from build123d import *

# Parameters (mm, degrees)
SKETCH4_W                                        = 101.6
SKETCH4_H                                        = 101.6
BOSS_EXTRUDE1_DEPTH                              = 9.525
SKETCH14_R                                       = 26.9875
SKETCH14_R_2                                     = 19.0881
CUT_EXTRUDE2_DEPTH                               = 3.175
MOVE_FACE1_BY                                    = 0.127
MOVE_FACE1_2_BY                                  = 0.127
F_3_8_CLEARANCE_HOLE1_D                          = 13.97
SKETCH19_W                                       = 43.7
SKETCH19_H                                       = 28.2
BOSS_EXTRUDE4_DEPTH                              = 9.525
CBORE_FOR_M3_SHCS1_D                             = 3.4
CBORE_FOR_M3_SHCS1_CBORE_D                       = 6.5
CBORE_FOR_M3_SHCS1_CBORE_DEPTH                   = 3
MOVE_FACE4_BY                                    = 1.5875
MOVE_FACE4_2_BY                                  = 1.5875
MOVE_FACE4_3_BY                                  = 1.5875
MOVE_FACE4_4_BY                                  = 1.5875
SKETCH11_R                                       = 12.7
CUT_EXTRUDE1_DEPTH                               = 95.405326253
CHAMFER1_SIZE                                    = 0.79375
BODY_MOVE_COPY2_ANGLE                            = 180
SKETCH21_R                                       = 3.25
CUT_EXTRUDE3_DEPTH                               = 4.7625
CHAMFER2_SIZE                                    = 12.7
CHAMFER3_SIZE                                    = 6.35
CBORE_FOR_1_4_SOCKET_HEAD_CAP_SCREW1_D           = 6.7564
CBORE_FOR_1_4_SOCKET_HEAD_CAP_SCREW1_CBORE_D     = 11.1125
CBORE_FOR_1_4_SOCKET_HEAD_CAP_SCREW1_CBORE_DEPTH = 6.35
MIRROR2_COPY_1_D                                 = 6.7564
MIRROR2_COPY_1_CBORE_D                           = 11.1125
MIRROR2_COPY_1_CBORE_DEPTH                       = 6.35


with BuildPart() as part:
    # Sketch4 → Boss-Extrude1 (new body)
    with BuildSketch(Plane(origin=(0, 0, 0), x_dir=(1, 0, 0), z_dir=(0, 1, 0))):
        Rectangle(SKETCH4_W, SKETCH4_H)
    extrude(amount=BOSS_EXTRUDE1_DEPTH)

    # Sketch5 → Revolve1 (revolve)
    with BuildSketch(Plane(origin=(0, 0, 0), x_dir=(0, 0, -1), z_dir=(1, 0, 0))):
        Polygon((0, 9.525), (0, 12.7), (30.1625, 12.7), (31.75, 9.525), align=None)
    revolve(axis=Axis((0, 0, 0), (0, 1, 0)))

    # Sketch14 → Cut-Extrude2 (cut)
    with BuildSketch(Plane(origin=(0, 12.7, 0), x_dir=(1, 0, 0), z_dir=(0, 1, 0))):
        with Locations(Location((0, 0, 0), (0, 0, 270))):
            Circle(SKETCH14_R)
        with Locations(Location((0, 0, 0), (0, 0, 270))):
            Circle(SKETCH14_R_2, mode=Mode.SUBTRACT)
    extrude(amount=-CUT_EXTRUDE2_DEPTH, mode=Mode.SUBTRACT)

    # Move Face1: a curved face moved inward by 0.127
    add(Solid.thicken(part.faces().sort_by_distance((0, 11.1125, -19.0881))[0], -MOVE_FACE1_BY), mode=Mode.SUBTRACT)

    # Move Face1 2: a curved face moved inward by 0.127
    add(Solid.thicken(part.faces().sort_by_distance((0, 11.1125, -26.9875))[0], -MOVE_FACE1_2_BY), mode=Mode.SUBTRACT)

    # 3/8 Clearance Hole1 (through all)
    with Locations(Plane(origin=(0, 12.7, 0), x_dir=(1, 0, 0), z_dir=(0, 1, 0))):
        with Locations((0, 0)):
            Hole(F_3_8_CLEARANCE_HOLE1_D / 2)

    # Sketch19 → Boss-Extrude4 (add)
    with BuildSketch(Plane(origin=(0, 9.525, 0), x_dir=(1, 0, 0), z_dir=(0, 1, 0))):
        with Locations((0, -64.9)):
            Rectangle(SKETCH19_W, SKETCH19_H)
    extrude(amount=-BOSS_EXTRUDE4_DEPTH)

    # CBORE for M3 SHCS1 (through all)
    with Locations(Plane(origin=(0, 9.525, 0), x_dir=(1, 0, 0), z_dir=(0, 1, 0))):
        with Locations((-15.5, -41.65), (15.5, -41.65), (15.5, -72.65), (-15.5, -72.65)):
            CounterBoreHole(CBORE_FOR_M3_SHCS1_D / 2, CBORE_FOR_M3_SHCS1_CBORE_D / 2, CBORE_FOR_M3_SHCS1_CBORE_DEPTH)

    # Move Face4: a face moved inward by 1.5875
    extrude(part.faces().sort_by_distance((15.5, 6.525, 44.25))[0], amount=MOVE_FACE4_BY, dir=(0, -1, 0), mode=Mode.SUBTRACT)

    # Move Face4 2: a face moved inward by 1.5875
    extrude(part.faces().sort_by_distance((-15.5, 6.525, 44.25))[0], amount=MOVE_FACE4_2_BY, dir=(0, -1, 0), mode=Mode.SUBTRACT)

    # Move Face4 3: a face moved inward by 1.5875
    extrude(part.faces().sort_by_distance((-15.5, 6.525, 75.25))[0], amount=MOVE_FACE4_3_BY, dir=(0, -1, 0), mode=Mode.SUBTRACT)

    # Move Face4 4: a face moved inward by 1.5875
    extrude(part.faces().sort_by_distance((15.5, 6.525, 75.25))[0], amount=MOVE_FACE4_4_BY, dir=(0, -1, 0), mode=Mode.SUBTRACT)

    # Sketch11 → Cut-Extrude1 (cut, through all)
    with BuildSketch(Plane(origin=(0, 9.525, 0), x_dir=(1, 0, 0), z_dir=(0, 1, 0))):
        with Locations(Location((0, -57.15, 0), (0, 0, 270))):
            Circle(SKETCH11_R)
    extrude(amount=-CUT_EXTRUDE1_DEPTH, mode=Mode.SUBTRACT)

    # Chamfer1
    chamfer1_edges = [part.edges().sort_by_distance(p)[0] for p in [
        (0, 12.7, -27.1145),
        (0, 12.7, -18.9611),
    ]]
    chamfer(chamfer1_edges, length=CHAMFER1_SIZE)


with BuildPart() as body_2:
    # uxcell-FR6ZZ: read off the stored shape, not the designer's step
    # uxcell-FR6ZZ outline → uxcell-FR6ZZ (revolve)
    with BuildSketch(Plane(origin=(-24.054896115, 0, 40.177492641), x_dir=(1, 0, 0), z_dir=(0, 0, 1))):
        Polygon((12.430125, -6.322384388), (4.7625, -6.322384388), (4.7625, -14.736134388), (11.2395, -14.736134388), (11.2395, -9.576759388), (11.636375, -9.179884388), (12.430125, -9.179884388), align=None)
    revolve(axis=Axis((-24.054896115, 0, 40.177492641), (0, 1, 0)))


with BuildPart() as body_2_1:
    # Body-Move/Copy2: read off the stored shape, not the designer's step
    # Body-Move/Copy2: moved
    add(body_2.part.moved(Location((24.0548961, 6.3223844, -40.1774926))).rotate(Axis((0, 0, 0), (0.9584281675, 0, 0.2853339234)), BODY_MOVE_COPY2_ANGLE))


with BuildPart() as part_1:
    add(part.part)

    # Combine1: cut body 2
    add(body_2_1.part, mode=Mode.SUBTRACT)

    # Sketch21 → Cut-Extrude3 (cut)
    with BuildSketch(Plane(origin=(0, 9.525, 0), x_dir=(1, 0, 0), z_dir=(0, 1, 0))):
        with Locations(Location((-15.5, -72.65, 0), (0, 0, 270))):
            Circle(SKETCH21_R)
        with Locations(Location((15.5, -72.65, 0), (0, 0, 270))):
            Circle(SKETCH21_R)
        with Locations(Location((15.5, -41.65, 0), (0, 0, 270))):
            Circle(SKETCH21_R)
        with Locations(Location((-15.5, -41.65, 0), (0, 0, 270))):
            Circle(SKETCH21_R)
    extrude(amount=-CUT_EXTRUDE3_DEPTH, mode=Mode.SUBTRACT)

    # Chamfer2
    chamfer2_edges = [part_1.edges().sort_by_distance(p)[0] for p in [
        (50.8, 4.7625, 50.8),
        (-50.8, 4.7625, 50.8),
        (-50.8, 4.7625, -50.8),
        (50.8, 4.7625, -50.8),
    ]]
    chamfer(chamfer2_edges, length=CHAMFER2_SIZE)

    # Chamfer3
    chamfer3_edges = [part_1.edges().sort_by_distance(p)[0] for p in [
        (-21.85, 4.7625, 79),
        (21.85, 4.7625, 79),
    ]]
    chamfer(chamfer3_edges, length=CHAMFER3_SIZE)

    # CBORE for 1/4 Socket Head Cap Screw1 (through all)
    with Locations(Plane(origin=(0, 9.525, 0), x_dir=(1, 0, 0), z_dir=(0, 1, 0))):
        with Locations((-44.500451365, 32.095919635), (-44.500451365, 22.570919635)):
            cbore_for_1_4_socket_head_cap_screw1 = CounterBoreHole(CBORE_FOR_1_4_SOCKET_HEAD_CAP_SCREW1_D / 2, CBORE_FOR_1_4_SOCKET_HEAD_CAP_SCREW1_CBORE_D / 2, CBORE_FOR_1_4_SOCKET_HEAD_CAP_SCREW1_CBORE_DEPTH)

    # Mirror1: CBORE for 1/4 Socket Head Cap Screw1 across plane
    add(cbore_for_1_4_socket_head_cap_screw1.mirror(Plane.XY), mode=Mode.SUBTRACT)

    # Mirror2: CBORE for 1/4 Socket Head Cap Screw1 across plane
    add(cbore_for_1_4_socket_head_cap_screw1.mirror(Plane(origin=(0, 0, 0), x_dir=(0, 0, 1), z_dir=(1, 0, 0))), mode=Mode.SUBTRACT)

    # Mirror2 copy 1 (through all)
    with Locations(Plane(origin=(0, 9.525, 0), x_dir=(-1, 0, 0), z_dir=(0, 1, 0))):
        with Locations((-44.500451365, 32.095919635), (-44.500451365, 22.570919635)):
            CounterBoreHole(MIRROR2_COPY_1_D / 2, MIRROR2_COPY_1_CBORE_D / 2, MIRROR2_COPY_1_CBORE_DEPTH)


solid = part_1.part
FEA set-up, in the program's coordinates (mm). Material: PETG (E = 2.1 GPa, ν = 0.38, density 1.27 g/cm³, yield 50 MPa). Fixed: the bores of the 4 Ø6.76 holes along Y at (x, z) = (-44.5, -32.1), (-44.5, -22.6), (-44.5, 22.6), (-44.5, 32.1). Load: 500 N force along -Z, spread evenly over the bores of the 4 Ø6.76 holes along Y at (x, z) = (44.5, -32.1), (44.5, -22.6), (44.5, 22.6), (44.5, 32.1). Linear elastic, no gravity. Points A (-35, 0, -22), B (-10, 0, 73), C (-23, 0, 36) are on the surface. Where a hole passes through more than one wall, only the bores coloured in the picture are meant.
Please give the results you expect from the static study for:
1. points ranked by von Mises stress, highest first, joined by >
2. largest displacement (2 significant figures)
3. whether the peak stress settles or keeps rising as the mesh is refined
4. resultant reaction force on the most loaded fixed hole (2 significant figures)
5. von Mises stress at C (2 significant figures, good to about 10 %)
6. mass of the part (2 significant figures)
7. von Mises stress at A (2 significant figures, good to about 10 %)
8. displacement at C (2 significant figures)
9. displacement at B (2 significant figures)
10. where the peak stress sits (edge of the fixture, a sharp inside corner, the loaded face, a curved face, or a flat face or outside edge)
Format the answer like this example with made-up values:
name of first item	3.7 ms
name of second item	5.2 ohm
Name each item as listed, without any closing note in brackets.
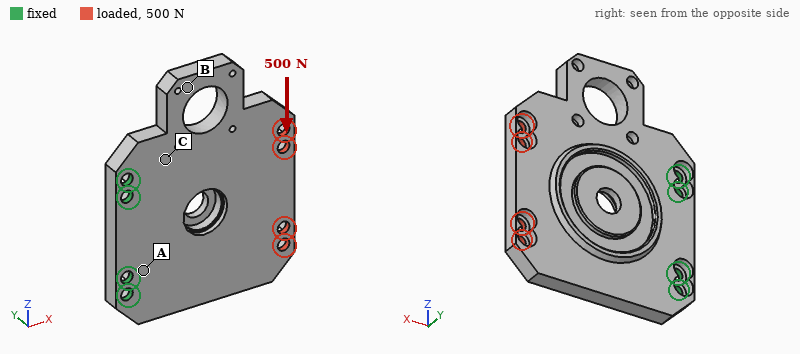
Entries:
points ranked by von Mises stress, highest first, joined by >	A > C > B
largest displacement	0.78 mm
whether the peak stress settles or keeps rising as the mesh is refined	keeps rising
resultant reaction force on the most loaded fixed hole	510 N
von Mises stress at C	3.7 MPa
mass of the part	120 g
von Mises stress at A	6.5 MPa
displacement at C	0.19 mm
displacement at B	0.54 mm
where the peak stress sits	edge of the fixture
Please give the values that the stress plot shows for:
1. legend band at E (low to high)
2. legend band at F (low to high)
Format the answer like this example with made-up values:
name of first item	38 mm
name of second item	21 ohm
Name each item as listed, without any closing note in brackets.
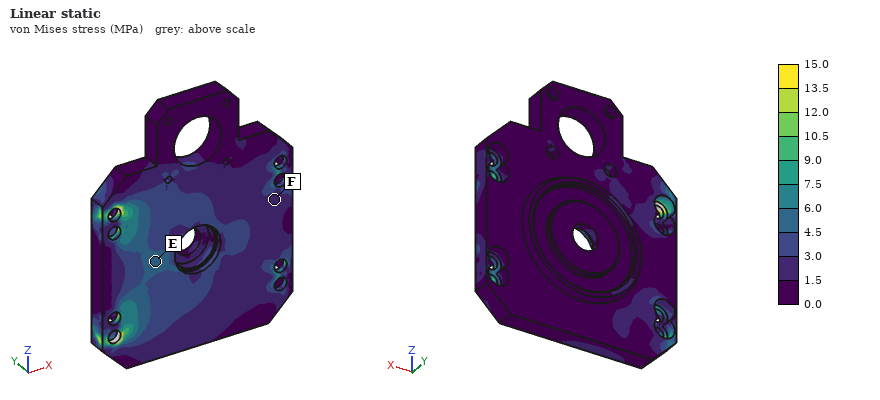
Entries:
legend band at E	4.5 to 6.0 MPa
legend band at F	1.5 to 3.0 MPa
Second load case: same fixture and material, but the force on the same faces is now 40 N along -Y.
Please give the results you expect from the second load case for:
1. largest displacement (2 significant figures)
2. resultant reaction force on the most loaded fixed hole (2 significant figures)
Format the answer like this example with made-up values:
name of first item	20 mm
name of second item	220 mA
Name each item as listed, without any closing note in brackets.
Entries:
largest displacement	1.6 mm
resultant reaction force on the most loaded fixed hole	26 N
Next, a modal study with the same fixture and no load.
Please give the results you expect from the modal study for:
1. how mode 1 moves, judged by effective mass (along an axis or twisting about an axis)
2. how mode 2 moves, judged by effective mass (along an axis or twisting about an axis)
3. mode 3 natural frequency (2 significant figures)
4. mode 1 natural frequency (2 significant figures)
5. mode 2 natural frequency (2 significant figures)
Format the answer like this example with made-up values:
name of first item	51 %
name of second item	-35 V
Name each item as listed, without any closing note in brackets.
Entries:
how mode 1 moves, judged by effective mass	along Y
how mode 2 moves, judged by effective mass	twisting about X
mode 3 natural frequency	790 Hz
mode 1 natural frequency	140 Hz
mode 2 natural frequency	370 Hz
